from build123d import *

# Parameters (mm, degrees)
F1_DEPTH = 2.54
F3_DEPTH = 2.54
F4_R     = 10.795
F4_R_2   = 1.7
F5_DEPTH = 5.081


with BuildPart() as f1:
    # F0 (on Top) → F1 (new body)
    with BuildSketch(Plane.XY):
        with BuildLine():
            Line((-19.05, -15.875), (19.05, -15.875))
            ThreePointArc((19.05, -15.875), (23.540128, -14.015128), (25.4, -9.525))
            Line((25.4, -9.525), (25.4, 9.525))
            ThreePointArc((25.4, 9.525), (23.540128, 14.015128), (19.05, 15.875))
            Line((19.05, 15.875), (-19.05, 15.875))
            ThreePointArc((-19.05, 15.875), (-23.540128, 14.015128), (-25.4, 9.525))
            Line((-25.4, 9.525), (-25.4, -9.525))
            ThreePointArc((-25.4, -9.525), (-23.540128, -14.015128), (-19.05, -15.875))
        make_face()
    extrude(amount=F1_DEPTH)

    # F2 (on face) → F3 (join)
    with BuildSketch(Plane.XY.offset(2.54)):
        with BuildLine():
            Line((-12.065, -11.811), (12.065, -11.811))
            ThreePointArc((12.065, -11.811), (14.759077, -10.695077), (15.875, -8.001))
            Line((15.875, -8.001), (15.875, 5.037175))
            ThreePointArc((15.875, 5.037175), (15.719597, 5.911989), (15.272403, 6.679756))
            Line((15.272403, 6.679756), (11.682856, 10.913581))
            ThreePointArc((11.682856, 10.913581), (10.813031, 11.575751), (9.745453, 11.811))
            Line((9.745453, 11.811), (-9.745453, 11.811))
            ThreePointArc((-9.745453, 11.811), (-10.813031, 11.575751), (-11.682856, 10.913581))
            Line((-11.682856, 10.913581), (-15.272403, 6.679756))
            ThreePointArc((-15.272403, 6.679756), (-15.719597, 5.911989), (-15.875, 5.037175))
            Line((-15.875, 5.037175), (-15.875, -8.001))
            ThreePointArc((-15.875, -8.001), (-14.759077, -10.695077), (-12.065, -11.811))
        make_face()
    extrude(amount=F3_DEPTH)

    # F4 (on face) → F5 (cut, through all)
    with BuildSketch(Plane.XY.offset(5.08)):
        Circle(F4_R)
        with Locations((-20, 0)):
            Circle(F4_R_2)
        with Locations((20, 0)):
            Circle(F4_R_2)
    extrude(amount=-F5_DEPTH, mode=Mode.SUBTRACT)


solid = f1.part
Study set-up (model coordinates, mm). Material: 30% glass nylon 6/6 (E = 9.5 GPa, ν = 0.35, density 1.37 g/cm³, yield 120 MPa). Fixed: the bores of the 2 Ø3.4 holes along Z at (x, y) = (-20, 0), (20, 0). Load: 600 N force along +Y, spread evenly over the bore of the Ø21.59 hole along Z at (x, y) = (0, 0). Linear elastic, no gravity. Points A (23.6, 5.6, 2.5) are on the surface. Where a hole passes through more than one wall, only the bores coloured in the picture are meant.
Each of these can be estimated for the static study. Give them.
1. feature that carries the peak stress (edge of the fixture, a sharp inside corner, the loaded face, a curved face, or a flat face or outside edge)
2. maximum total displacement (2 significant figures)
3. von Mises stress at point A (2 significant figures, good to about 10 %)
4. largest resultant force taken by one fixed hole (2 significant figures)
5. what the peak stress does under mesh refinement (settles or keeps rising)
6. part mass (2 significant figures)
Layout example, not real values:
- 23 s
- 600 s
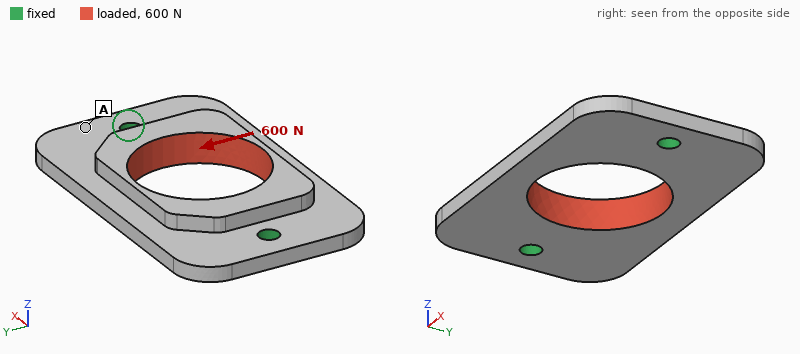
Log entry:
- edge of the fixture
- 84 µm
- 6.1 MPa
- 300 N
- keeps rising
- 5.4 g
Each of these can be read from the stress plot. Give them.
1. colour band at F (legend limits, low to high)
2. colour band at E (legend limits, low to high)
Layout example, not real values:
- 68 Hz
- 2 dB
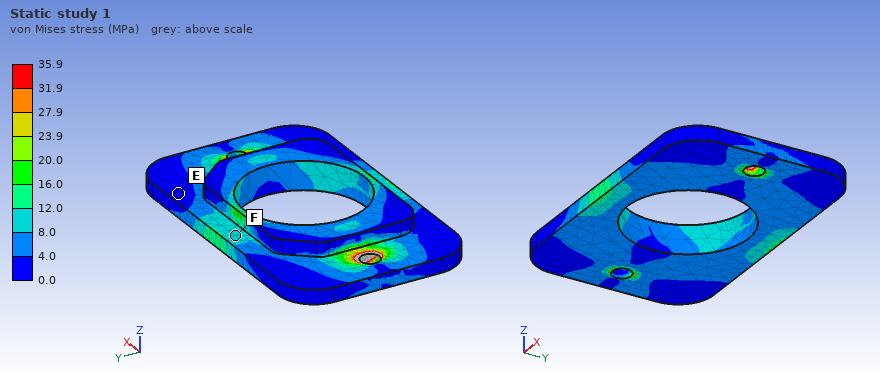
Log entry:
- 8.0 to 12.0 MPa
- 0.0 to 4.0 MPa
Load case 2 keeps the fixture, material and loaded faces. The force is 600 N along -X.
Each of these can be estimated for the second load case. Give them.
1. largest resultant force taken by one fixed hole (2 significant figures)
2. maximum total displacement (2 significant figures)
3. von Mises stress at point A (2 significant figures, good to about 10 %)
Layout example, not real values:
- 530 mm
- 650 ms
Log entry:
- 300 N
- 20 µm
- 3.8 MPa
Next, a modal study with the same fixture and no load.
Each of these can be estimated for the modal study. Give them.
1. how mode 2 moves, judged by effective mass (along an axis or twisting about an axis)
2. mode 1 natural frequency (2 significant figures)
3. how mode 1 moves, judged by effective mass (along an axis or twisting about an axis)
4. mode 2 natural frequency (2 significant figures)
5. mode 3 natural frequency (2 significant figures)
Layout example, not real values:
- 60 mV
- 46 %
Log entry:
- along Z
- 3000 Hz
- twisting about X
- 4200 Hz
- 5700 Hz
